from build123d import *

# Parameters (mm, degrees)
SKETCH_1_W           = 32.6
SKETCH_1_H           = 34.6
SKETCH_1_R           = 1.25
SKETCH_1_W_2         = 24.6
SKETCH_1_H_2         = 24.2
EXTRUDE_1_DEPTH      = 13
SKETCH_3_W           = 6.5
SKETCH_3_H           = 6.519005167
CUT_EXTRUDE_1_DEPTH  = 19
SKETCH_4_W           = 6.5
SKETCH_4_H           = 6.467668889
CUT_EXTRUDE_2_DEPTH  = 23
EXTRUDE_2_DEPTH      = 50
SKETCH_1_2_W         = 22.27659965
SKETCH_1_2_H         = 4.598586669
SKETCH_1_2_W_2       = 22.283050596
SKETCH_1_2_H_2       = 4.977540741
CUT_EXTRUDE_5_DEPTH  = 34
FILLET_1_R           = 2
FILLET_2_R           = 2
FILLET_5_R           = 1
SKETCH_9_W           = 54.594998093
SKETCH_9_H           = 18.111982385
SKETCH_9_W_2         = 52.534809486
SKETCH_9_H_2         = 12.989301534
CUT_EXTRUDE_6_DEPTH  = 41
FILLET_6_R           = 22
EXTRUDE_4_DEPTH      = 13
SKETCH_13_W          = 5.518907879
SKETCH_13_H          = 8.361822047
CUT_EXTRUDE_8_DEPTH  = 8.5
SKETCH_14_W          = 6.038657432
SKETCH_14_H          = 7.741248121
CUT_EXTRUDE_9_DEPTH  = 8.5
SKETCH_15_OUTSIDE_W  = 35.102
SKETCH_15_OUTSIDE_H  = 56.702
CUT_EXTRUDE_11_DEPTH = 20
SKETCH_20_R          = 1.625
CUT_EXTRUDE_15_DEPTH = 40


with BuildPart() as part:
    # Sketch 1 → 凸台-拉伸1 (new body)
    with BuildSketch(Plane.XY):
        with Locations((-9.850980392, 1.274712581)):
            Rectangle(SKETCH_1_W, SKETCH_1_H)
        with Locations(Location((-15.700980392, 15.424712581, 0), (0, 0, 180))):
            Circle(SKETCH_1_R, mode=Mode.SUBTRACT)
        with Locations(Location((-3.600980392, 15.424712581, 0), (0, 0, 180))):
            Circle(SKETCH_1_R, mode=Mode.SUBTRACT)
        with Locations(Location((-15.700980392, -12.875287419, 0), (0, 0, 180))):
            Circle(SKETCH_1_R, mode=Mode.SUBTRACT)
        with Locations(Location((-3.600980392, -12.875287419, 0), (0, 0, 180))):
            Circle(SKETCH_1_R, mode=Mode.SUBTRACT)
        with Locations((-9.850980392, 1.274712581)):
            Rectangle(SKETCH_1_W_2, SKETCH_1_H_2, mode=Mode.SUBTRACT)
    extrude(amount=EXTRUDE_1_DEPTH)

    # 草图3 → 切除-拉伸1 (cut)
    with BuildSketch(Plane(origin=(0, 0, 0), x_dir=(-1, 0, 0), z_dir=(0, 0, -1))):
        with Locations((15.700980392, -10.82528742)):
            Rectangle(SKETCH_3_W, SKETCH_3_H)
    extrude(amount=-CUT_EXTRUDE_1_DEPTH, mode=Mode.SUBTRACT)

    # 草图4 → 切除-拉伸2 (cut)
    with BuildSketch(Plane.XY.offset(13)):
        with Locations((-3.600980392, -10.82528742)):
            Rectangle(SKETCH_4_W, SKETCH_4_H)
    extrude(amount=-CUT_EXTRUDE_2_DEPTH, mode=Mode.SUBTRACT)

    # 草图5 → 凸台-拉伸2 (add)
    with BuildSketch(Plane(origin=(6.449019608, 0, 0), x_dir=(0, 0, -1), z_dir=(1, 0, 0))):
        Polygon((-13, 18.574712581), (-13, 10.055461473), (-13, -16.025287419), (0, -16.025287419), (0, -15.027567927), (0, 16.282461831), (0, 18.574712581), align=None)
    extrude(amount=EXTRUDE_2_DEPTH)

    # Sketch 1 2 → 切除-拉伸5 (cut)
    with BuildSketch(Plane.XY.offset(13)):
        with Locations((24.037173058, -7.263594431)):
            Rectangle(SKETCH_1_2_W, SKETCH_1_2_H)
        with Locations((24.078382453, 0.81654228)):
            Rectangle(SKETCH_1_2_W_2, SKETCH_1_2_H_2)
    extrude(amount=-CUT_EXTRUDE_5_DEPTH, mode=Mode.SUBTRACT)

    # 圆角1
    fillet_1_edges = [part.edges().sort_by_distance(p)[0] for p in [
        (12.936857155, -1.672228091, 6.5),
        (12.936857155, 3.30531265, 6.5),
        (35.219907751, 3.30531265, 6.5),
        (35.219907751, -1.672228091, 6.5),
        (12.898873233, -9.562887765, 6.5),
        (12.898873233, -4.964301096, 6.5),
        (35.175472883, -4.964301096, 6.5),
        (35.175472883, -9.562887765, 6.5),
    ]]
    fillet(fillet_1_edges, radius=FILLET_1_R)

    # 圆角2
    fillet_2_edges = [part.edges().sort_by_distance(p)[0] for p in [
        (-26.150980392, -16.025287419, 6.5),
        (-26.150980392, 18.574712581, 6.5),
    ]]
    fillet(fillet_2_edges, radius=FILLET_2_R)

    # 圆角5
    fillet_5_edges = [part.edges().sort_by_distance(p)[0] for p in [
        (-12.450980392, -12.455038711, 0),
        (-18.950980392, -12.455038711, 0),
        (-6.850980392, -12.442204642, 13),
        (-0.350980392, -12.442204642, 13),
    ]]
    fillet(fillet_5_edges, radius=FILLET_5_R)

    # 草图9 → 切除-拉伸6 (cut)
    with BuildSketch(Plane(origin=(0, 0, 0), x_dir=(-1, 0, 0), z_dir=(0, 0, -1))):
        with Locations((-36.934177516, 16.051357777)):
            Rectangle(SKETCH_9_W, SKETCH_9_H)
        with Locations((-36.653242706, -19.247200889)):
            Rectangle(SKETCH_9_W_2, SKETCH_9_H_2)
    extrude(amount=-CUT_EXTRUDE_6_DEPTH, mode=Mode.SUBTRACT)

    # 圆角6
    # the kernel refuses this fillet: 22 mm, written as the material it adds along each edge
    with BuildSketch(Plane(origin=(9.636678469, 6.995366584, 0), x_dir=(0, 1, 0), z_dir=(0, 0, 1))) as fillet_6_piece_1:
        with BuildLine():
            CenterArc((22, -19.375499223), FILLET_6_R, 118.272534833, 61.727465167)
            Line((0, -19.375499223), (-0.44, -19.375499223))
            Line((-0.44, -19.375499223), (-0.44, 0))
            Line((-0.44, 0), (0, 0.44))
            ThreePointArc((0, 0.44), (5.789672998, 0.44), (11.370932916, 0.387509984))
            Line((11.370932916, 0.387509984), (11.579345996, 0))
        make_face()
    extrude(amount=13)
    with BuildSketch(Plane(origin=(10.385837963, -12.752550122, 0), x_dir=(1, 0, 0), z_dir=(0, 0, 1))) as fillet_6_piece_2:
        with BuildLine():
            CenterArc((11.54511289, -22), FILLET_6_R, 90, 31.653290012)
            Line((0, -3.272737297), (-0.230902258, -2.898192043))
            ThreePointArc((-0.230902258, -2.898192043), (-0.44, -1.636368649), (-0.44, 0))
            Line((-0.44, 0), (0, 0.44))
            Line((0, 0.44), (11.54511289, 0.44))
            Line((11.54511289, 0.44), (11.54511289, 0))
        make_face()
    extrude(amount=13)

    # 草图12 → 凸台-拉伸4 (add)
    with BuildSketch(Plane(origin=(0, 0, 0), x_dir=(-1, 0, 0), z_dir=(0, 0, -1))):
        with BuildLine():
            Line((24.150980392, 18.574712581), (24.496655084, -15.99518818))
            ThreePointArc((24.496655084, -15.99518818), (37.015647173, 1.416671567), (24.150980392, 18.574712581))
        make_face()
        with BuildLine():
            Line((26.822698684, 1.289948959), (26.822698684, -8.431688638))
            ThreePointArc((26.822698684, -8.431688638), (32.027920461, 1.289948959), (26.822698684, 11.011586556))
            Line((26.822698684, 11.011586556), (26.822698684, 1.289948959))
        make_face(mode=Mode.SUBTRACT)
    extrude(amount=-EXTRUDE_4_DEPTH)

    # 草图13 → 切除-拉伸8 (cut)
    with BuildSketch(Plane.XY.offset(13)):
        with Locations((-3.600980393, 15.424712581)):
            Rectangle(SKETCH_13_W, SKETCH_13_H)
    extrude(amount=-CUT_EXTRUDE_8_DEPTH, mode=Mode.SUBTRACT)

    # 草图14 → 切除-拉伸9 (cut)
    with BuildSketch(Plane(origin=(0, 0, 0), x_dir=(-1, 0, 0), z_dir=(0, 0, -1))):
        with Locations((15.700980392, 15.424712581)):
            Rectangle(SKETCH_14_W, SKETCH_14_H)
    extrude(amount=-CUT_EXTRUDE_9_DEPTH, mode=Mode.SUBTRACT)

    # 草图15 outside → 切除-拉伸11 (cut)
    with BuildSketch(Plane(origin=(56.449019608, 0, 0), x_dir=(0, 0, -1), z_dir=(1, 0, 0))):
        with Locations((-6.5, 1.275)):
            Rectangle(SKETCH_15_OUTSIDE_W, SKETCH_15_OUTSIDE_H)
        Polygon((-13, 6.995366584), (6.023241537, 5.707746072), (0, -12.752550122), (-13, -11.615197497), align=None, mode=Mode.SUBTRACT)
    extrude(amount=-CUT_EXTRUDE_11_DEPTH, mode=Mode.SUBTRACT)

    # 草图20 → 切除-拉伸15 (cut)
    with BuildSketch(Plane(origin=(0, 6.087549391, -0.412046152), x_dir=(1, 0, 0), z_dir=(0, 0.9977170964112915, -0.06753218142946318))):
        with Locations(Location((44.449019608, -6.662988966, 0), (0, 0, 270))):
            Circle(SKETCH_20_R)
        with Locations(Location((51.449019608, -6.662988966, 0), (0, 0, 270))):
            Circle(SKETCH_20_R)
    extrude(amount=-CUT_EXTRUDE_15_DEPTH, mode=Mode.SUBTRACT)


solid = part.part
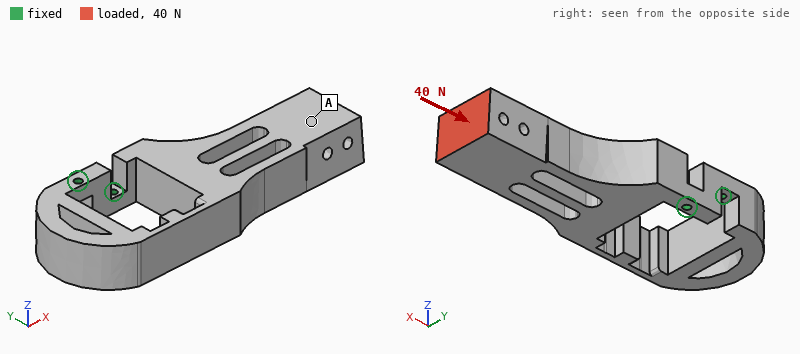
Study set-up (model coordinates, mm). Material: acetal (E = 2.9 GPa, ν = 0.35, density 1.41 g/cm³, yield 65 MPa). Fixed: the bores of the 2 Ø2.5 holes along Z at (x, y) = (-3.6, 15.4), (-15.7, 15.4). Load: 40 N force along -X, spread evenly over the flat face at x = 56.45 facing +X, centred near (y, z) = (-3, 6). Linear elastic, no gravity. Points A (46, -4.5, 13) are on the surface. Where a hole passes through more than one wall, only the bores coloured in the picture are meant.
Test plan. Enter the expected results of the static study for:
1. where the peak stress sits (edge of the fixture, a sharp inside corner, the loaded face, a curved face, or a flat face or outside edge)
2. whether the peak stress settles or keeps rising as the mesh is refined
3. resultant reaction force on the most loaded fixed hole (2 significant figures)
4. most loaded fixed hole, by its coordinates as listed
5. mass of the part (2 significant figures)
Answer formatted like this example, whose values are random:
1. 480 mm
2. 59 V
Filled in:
1. edge of the fixture
2. keeps rising
3. 32 N
4. (-3.6, 15.4)
5. 27 g
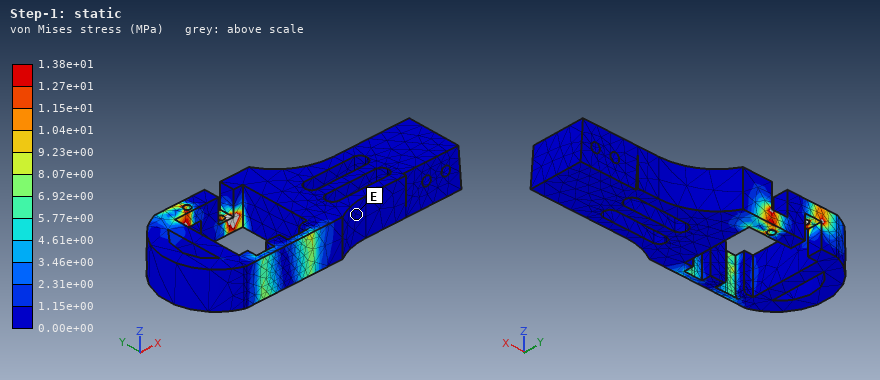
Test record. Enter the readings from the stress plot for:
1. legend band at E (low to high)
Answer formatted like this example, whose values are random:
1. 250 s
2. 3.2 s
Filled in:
1. 0.00e+00 to 1.15e+00 MPa
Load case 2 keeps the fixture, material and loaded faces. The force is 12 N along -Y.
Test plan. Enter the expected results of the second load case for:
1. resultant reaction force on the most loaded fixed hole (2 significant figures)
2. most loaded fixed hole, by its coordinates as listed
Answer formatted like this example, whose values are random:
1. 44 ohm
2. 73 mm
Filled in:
1. 27 N
2. (-3.6, 15.4)
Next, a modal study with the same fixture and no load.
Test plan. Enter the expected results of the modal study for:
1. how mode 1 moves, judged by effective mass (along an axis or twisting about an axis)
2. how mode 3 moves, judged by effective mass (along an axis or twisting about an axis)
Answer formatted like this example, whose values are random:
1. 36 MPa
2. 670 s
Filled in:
1. along Z
2. along Z
